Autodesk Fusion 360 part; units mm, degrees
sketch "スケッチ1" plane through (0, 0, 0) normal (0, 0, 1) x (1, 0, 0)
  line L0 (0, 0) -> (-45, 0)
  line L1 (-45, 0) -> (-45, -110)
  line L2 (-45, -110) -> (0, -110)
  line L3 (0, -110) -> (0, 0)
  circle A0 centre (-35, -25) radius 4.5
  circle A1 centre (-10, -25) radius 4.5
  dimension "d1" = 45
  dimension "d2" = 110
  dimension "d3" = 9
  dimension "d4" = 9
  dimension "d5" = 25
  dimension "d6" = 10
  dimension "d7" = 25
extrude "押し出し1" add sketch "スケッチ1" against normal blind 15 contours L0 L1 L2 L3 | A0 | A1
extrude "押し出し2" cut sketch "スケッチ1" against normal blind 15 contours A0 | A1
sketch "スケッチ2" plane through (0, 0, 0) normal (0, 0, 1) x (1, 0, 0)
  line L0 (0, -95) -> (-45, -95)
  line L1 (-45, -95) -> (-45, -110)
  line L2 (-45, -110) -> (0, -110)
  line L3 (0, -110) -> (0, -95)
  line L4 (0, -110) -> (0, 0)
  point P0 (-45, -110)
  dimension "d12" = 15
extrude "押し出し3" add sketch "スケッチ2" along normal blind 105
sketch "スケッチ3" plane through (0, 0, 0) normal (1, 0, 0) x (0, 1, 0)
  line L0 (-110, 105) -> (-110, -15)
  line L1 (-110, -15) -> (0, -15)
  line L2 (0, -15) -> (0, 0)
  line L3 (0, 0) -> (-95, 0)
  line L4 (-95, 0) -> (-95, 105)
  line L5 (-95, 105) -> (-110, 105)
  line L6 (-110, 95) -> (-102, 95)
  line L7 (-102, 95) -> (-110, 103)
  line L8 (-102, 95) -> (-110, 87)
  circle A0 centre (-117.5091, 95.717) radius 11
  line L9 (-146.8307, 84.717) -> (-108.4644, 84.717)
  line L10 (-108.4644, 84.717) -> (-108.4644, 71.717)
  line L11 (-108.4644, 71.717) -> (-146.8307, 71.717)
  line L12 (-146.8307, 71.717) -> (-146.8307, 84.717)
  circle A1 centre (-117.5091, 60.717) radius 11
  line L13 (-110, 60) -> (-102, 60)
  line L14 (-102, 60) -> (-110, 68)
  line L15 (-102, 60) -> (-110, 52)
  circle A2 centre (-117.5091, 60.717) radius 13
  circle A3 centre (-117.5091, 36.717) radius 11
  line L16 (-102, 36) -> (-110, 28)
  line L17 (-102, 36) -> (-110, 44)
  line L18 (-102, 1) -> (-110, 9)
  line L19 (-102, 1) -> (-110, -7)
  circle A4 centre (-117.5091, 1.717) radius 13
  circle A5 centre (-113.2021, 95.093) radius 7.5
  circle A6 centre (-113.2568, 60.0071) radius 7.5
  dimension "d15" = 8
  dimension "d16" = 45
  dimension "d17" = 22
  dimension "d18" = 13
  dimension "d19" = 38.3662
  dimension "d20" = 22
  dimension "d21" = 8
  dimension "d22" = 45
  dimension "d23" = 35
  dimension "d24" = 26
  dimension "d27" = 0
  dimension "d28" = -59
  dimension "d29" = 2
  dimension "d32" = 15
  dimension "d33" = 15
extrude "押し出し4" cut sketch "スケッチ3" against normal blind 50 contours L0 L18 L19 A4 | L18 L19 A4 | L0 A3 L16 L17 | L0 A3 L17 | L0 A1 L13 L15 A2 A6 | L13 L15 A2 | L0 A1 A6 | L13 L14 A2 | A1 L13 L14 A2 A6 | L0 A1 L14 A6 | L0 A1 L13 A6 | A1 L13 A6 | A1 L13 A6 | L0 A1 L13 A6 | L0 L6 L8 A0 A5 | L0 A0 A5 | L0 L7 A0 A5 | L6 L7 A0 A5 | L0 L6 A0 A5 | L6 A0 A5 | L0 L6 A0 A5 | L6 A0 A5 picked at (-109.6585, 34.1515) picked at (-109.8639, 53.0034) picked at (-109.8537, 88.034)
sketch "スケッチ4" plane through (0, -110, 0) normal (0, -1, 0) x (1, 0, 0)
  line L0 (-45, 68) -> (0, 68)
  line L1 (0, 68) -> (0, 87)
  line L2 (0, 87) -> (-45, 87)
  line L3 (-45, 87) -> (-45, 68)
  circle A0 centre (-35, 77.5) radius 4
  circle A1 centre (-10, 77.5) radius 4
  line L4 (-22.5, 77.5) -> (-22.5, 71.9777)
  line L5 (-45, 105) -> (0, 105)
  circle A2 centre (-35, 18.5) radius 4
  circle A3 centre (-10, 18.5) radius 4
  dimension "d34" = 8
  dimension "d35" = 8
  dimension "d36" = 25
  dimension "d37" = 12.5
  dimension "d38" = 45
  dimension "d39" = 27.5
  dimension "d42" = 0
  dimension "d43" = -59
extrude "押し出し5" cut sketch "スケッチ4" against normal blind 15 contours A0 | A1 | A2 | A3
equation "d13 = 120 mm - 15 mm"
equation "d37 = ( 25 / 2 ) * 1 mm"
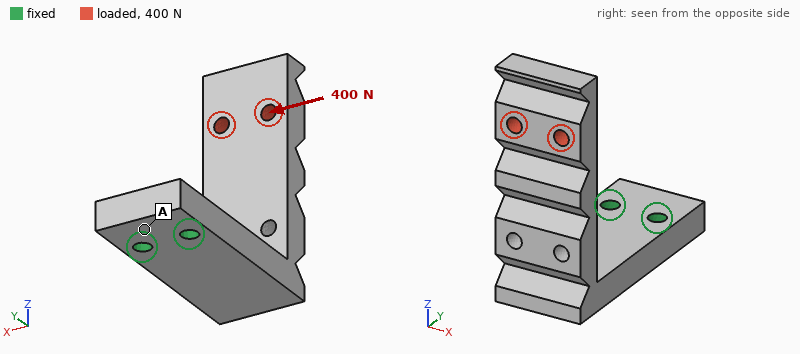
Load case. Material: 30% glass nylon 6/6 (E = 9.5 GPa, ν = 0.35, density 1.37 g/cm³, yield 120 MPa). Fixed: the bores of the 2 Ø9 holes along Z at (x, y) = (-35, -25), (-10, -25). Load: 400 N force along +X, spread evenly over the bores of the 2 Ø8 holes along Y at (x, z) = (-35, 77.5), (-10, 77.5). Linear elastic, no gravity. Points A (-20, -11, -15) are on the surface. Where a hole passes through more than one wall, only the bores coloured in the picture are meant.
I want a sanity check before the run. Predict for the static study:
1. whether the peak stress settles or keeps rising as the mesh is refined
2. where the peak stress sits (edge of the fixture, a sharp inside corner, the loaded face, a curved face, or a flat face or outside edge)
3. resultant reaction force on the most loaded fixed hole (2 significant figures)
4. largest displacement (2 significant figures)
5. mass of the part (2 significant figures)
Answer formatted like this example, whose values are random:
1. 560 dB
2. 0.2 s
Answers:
1. keeps rising
2. edge of the fixture
3. 1.4 kN
4. 1.9 mm
5. 180 g
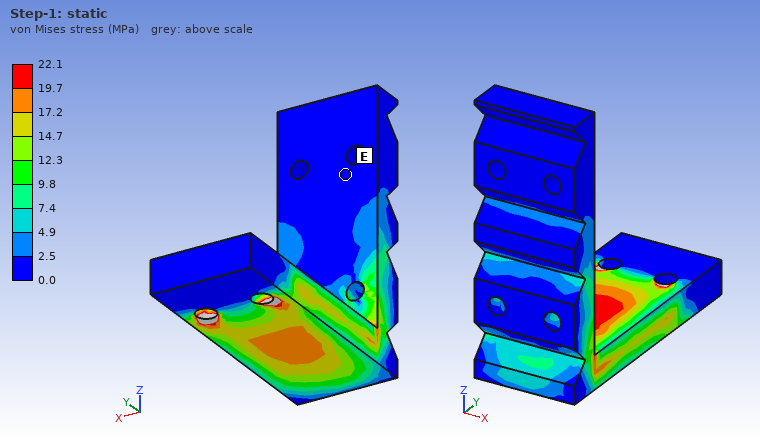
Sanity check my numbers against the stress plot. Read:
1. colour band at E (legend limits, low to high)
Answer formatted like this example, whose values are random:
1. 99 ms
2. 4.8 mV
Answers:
1. 0.0 to 2.5 MPa
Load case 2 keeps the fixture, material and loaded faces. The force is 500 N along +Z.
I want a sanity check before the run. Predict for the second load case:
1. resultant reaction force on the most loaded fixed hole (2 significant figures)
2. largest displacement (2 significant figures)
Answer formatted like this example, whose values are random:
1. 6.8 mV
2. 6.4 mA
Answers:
1. 250 N
2. 1.7 mm
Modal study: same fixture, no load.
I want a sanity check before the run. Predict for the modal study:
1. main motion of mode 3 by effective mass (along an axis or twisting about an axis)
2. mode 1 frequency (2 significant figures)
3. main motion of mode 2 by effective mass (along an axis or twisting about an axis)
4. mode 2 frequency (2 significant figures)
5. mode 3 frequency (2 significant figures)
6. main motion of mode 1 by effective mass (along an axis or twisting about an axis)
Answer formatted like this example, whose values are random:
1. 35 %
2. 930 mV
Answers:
1. along Z
2. 230 Hz
3. along X
4. 370 Hz
5. 610 Hz
6. along Y
